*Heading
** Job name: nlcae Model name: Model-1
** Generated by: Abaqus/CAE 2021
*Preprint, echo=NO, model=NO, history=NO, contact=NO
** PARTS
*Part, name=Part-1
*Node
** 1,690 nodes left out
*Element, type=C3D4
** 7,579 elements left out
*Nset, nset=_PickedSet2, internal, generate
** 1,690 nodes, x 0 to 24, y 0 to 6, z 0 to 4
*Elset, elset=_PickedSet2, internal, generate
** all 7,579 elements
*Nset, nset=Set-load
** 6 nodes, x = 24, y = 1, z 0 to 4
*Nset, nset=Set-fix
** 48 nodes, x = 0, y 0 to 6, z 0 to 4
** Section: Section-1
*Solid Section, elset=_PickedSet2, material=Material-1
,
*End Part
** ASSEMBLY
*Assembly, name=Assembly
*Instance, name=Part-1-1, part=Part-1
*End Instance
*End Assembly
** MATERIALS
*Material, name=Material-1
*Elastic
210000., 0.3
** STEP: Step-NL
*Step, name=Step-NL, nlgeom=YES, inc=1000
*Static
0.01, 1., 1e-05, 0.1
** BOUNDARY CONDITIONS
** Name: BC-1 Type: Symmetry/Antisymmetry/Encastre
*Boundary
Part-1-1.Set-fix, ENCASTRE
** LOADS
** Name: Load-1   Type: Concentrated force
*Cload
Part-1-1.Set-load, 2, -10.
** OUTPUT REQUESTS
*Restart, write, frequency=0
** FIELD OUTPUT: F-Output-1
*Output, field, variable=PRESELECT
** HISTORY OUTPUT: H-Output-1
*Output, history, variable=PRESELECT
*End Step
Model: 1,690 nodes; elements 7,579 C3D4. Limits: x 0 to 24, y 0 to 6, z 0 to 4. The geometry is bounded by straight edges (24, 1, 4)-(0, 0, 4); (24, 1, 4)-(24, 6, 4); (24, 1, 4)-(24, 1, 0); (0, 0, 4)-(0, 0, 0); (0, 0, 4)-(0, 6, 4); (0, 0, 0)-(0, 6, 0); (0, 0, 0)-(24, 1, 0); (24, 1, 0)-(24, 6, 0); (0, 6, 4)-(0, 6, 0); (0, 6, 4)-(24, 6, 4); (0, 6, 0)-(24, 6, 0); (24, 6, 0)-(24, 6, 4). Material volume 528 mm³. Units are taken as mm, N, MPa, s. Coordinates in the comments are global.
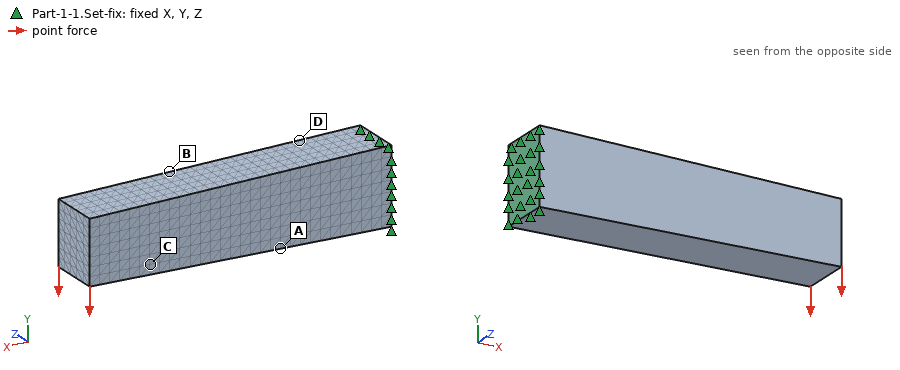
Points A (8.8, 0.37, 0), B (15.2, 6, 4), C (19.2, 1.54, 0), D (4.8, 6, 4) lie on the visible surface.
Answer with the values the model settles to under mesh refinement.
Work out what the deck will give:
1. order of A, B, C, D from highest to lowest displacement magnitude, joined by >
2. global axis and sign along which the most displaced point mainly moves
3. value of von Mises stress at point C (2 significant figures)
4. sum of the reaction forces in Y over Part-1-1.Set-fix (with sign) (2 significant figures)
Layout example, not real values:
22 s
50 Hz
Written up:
C > B > A > D
-Y
12 MPa
60 N
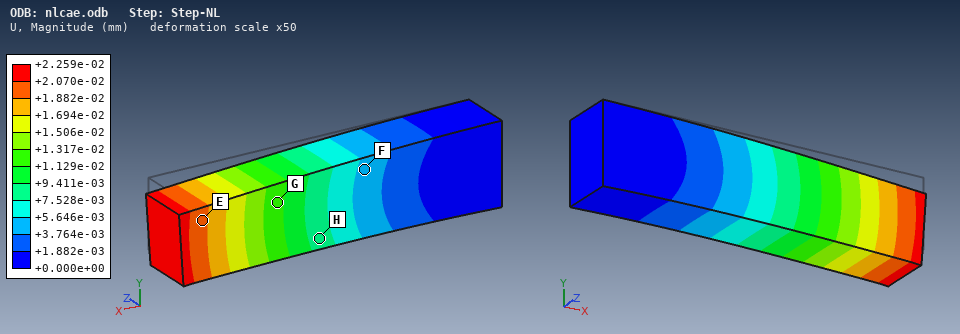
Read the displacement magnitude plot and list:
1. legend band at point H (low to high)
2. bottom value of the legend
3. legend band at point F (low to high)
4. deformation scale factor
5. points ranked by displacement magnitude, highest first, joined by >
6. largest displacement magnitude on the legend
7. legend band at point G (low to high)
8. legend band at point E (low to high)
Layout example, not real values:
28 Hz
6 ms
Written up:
+7.528e-03 to +9.411e-03 mm
+0.000e+00 mm
+3.764e-03 to +5.646e-03 mm
50
E > G > H > F
+2.259e-02 mm
+1.129e-02 to +1.317e-02 mm
+1.882e-02 to +2.070e-02 mm
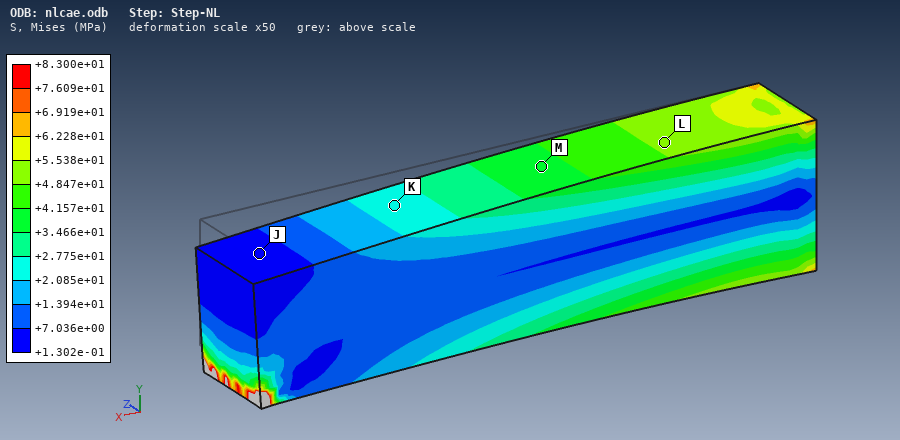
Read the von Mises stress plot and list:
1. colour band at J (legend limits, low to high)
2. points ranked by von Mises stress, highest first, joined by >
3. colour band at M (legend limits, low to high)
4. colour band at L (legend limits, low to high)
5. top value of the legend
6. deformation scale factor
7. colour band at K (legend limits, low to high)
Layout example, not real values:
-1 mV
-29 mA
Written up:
+1.302e-01 to +7.036e+00 MPa
L > M > K > J
+3.466e+01 to +4.157e+01 MPa
+4.847e+01 to +5.538e+01 MPa
+8.300e+01 MPa
50
+2.085e+01 to +2.775e+01 MPa
